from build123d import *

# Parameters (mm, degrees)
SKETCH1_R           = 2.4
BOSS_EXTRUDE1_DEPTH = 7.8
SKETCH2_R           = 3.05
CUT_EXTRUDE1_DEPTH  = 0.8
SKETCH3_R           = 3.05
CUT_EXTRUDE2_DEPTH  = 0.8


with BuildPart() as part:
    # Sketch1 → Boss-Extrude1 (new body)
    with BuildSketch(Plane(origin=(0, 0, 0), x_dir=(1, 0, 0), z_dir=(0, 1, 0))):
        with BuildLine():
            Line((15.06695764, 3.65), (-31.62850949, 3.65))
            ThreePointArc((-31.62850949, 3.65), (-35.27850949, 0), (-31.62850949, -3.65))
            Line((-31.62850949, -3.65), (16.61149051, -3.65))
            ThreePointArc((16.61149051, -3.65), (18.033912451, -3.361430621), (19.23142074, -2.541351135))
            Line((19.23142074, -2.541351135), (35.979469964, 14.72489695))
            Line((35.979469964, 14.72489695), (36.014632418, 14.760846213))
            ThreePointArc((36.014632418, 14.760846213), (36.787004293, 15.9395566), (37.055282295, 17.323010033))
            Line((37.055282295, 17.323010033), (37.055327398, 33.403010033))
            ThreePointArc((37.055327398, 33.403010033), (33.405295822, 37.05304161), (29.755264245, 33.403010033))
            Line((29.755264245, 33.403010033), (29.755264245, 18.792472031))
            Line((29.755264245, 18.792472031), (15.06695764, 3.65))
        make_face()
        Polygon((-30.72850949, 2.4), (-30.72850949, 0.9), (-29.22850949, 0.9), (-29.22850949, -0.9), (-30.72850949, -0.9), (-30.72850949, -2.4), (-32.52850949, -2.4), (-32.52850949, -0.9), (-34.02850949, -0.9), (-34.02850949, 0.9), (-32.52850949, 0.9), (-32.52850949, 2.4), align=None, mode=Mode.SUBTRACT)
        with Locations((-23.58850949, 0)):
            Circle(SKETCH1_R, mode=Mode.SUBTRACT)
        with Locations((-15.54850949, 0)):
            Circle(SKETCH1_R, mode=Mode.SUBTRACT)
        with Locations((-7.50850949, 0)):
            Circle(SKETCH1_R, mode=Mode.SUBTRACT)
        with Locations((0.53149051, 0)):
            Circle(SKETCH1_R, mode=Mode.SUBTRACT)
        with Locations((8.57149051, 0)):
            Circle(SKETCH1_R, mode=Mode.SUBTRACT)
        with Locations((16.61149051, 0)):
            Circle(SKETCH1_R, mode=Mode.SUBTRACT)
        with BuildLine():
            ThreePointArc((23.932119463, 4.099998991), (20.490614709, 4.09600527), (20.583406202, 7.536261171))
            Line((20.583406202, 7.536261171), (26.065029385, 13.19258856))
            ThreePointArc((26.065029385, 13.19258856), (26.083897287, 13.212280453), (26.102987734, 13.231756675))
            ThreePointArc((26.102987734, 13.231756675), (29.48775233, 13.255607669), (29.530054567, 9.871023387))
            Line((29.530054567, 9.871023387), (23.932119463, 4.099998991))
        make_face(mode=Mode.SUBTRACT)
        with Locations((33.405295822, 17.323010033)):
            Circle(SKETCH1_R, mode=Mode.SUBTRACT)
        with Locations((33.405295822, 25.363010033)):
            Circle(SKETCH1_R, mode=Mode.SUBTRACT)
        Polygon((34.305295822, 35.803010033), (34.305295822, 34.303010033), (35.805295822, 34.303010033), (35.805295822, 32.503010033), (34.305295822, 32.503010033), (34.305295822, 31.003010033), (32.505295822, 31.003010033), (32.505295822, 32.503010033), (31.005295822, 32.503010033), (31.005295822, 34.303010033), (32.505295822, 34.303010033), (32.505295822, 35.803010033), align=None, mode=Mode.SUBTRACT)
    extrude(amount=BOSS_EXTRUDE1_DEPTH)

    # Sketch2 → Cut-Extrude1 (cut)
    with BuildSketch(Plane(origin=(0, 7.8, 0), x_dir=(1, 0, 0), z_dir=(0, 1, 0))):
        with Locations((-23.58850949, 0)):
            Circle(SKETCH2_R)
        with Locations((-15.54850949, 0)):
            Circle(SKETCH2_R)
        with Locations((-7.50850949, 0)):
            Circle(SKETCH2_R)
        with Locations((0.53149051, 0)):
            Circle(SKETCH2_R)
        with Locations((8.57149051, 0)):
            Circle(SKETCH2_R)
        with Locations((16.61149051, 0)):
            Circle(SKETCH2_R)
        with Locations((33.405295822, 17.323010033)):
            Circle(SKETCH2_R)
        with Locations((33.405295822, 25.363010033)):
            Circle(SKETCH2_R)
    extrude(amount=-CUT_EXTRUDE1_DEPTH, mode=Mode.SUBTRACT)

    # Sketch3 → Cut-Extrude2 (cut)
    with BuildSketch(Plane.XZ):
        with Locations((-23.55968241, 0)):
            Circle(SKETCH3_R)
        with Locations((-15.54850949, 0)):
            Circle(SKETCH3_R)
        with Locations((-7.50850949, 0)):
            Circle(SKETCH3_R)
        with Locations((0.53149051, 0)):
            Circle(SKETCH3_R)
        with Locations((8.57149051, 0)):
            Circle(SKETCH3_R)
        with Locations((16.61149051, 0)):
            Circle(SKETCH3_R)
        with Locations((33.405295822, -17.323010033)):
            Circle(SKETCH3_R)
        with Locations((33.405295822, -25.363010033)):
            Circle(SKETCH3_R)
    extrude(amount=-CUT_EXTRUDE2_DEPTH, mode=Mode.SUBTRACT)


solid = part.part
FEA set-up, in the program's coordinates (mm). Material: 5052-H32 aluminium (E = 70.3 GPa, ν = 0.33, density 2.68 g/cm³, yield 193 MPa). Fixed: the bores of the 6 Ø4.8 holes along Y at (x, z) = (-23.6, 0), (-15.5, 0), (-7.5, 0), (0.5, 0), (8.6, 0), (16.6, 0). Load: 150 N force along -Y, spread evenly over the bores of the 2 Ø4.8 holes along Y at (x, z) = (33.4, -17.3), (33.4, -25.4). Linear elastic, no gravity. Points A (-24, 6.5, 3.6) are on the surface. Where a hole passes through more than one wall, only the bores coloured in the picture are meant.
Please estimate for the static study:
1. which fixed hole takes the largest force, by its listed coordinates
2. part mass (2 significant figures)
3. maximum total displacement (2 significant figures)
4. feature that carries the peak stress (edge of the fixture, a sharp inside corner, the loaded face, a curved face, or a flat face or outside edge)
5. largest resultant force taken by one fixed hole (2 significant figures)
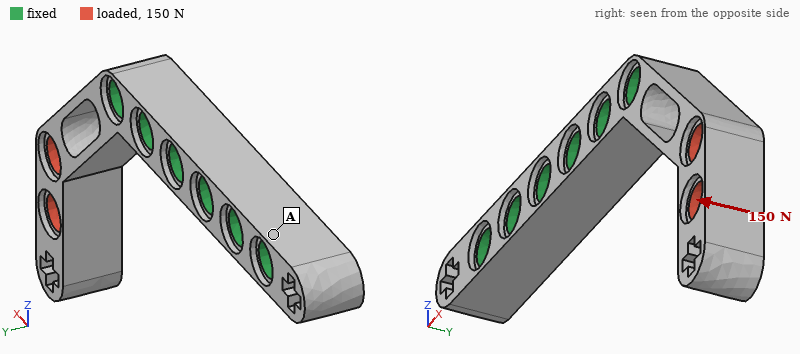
(16.6, 0)
9.2 g
0.22 mm
a curved face
180 N
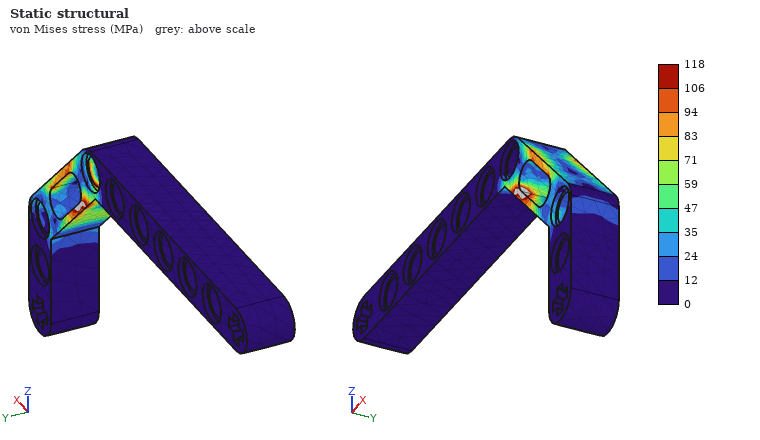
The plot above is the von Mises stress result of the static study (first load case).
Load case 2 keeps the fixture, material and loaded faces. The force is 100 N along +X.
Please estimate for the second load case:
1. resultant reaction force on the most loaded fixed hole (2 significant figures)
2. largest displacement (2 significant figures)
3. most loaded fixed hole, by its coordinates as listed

69 N
0.12 mm
(8.6, 0)
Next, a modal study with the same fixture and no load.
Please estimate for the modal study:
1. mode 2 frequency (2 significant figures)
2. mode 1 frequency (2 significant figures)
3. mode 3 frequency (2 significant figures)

2700 Hz
2700 Hz
8400 Hz
